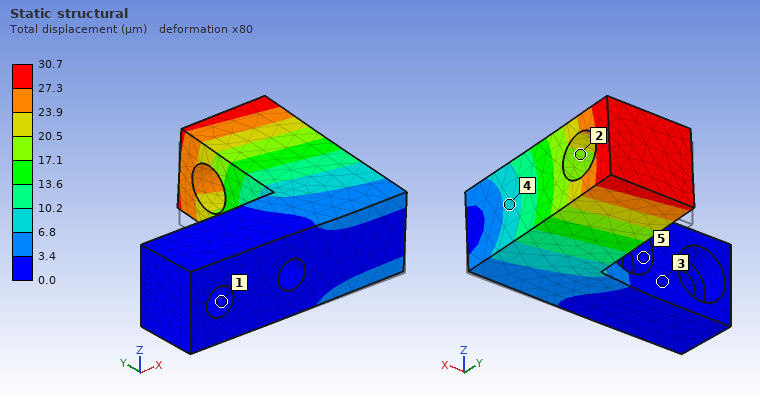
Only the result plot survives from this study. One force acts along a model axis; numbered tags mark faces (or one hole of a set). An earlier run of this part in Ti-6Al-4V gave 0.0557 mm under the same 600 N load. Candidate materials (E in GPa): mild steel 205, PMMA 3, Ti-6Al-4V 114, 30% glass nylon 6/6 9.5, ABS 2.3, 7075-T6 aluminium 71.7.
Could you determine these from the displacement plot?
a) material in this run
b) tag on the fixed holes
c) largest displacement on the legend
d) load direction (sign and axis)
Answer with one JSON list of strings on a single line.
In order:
["mild steel", "1", "30.7 µm", "+Z"]
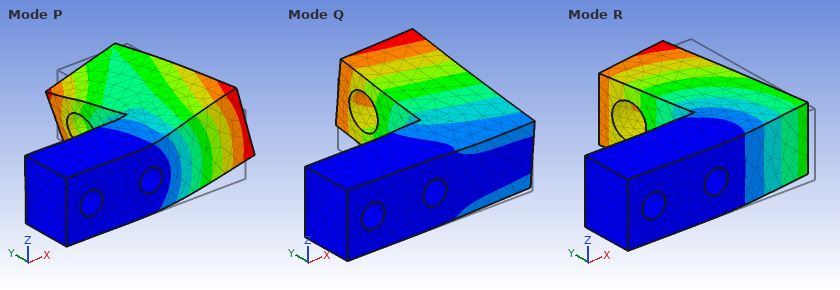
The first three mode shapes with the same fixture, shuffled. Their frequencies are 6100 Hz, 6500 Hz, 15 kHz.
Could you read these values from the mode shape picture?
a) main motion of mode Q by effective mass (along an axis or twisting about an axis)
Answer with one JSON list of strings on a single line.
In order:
["along Z"]
